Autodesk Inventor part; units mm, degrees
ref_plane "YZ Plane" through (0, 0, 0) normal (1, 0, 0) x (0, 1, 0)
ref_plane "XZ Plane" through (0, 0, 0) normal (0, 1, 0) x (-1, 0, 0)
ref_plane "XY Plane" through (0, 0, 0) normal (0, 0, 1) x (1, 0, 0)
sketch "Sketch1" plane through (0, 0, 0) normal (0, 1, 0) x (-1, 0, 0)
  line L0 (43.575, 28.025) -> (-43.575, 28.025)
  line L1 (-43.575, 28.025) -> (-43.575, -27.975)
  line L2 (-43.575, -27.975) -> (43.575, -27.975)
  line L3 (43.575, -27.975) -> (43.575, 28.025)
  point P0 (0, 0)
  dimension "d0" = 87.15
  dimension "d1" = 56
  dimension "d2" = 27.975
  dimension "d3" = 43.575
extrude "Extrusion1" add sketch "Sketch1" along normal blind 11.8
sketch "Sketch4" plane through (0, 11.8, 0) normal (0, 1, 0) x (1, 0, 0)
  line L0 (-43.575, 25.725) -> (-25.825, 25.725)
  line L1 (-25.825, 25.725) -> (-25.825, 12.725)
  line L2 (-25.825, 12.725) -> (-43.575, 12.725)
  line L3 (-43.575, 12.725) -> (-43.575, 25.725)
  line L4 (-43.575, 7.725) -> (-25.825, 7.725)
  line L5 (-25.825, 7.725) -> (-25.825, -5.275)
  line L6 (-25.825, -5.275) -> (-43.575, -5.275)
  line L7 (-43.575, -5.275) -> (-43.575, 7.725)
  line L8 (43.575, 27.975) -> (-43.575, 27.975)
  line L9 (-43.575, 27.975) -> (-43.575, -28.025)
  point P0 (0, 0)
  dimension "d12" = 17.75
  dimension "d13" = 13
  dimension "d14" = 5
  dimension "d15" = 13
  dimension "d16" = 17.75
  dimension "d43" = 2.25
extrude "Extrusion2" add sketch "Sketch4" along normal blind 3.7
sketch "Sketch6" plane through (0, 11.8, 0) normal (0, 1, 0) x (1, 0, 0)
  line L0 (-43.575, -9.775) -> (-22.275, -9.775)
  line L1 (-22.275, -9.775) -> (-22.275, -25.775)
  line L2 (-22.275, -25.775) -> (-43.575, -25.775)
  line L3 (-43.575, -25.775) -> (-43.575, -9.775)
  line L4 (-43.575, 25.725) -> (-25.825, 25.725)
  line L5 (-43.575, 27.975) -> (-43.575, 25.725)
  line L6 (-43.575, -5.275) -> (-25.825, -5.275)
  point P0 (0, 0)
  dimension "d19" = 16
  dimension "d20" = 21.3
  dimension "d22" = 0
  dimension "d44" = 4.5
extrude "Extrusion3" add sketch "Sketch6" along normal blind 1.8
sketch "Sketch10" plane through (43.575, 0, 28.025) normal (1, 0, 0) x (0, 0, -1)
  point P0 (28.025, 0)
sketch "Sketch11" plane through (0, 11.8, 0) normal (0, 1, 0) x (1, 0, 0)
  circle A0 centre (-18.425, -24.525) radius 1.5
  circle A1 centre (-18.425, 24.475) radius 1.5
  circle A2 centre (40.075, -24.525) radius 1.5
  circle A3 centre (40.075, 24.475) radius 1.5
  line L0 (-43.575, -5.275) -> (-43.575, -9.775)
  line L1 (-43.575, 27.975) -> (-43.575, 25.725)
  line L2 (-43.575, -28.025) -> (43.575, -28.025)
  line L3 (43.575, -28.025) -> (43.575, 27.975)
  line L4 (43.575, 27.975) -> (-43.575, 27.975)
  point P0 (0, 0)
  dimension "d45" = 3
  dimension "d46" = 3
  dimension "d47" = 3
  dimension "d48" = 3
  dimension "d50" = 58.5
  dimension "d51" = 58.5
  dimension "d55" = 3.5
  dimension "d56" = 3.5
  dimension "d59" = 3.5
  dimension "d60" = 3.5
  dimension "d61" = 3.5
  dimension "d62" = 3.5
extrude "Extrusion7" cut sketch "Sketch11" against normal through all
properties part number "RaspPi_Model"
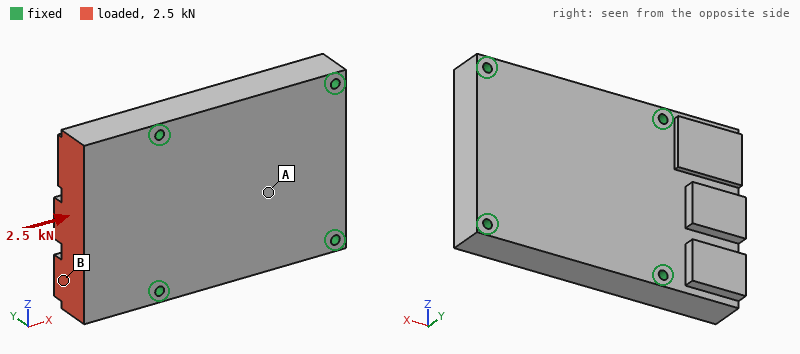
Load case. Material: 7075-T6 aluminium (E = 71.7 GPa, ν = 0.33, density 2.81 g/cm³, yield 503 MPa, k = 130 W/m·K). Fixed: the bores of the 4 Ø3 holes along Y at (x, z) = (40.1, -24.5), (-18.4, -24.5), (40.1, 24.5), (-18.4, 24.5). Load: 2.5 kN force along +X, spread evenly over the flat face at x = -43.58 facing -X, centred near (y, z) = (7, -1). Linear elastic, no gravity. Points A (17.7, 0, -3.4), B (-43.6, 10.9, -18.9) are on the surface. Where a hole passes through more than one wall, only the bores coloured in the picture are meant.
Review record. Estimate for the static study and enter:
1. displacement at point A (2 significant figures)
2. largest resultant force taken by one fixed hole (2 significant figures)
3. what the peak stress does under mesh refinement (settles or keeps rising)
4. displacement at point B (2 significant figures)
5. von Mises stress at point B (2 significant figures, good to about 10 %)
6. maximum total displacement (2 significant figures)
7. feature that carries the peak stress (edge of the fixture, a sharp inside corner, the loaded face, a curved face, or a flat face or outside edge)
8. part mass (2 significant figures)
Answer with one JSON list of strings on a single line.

["0.61 µm", "1.1 kN", "keeps rising", "3.2 µm", "3.1 MPa", "3.8 µm", "edge of the fixture", "170 g"]
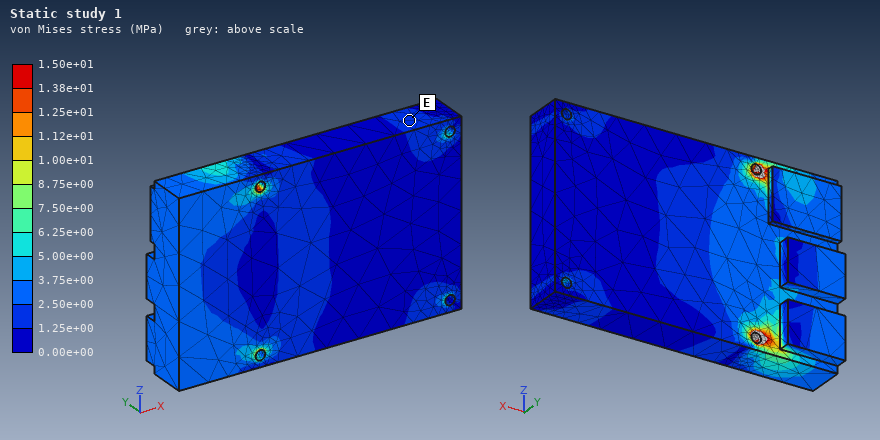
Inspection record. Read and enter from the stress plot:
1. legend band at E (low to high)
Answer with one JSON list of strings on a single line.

["1.25e+00 to 2.50e+00 MPa"]
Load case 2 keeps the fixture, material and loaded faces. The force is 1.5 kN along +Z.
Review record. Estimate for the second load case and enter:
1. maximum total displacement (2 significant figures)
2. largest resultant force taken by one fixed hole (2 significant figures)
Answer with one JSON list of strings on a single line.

["4.5 µm", "1.0 kN"]
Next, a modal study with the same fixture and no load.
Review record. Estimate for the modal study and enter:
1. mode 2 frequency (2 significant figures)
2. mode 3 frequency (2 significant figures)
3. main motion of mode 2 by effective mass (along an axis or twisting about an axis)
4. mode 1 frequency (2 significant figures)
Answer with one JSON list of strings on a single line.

["10 kHz", "15 kHz", "along Y", "8200 Hz"]
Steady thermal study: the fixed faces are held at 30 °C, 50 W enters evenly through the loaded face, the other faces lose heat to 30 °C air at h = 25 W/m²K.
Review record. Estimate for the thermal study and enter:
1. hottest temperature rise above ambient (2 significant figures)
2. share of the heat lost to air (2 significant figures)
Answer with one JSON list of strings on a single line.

["18 K", "3.2 %"]
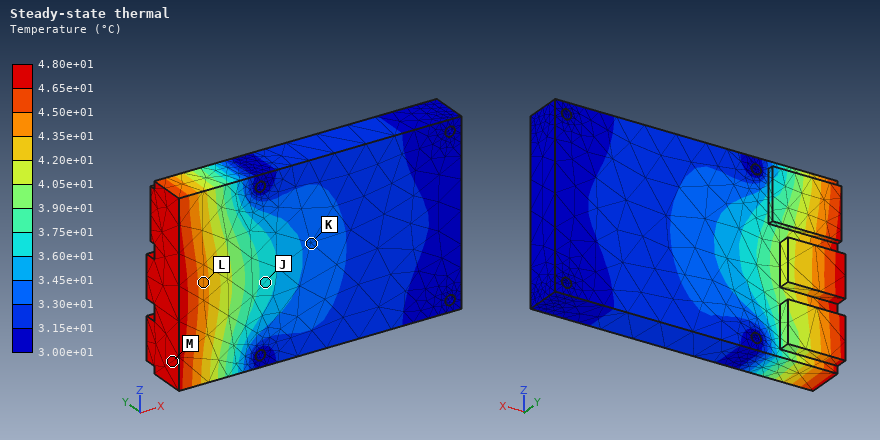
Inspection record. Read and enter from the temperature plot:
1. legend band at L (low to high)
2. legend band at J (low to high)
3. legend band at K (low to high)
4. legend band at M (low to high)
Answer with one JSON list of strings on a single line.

["4.35e+01 to 4.50e+01 °C", "3.60e+01 to 3.75e+01 °C", "3.30e+01 to 3.45e+01 °C", "4.65e+01 to 4.80e+01 °C"]
